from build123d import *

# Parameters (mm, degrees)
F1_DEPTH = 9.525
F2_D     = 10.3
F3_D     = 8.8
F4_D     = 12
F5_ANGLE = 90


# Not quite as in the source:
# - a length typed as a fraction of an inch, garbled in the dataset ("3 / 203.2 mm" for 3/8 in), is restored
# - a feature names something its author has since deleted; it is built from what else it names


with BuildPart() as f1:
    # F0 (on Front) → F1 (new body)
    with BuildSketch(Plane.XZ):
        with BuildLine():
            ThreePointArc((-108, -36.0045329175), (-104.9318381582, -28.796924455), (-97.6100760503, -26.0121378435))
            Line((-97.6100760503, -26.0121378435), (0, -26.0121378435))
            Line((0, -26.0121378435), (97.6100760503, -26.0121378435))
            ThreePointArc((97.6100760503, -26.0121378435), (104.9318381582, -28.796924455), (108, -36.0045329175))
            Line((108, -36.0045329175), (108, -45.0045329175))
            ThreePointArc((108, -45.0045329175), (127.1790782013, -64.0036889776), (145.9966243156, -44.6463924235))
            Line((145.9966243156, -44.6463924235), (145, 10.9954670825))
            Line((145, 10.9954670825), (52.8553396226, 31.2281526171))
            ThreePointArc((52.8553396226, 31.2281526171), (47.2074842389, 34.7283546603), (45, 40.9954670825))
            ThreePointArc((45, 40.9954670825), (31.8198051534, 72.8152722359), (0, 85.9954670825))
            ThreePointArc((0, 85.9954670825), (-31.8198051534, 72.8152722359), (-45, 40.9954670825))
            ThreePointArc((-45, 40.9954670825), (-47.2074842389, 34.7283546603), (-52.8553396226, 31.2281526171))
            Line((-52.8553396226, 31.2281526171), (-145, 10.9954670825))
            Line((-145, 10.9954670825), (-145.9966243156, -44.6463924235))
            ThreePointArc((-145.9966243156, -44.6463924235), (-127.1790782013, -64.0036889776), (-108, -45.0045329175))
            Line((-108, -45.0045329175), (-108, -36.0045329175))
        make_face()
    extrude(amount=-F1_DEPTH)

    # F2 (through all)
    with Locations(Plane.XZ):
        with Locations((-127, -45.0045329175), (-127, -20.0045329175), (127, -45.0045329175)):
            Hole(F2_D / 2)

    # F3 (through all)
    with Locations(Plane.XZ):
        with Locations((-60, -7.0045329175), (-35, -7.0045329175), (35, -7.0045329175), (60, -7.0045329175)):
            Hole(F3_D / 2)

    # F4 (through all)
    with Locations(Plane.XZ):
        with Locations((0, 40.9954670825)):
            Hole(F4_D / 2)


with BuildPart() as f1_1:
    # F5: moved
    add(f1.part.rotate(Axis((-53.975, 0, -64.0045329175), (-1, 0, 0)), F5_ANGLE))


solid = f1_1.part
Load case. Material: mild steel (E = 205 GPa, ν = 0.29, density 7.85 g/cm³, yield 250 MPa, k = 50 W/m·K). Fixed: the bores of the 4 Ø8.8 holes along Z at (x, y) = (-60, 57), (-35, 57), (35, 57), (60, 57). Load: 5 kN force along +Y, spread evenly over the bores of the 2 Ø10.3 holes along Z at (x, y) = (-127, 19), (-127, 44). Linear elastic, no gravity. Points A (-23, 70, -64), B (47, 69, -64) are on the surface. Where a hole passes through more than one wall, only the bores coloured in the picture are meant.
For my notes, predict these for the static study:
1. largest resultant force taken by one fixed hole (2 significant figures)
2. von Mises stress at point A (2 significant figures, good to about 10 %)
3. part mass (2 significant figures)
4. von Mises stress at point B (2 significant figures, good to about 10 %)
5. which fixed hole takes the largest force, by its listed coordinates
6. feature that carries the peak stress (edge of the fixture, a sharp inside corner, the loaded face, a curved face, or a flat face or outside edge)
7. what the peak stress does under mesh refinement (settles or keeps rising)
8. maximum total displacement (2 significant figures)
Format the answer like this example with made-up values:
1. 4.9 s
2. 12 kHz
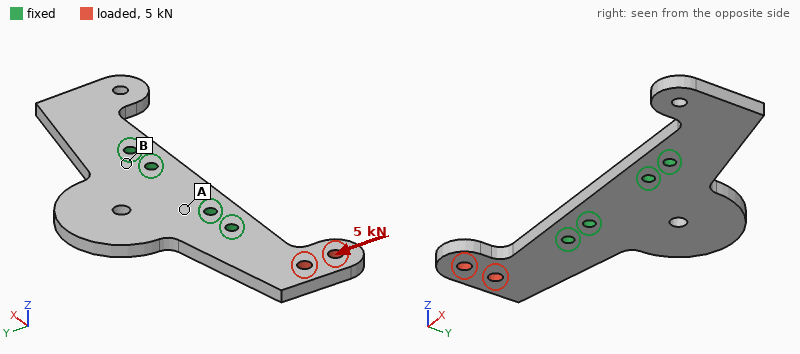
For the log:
1. 9.8 kN
2. 14 MPa
3. 1.6 kg
4. 6.3 MPa
5. (-60, 57)
6. edge of the fixture
7. keeps rising
8. 80 µm
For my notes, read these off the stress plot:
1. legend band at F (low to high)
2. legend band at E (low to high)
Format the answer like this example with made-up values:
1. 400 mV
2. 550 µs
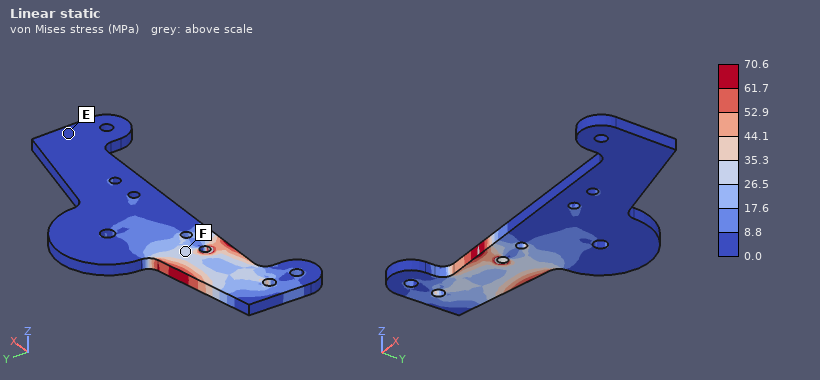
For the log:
1. 26.5 to 35.3 MPa
2. 0.0 to 8.8 MPa
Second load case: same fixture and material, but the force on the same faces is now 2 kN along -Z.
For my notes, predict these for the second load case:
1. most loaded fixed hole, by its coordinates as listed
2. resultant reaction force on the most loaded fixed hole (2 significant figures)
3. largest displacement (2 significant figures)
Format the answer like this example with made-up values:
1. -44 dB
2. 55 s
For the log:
1. (-60, 57)
2. 3.8 kN
3. 0.57 mm
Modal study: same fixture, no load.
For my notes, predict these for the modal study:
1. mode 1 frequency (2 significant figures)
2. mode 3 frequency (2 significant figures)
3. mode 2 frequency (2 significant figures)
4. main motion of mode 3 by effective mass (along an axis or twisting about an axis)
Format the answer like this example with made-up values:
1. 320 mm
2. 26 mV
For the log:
1. 840 Hz
2. 1200 Hz
3. 850 Hz
4. along Z
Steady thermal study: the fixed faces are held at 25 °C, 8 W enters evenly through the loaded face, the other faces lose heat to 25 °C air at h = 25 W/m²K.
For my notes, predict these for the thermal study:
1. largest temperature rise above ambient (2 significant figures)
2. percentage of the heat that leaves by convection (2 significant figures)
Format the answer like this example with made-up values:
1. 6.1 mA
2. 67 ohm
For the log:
1. 21 K
2. 45 %
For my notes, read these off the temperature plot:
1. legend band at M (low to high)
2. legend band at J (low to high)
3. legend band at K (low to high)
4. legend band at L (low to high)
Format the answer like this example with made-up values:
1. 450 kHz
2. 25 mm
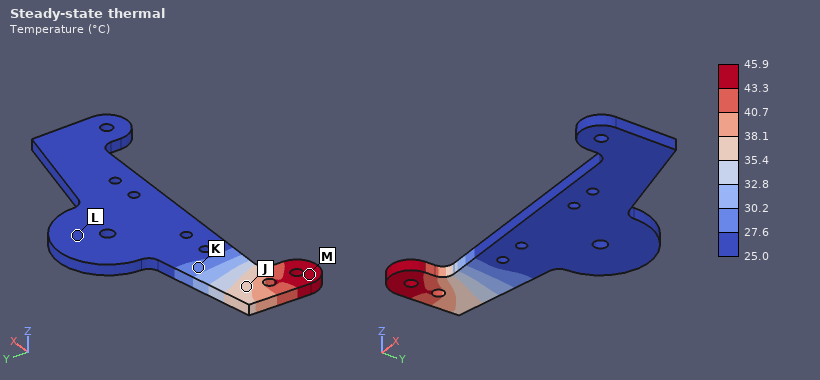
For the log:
1. 43.3 to 45.9 °C
2. 35.4 to 38.1 °C
3. 27.6 to 30.2 °C
4. 25.0 to 27.6 °C
